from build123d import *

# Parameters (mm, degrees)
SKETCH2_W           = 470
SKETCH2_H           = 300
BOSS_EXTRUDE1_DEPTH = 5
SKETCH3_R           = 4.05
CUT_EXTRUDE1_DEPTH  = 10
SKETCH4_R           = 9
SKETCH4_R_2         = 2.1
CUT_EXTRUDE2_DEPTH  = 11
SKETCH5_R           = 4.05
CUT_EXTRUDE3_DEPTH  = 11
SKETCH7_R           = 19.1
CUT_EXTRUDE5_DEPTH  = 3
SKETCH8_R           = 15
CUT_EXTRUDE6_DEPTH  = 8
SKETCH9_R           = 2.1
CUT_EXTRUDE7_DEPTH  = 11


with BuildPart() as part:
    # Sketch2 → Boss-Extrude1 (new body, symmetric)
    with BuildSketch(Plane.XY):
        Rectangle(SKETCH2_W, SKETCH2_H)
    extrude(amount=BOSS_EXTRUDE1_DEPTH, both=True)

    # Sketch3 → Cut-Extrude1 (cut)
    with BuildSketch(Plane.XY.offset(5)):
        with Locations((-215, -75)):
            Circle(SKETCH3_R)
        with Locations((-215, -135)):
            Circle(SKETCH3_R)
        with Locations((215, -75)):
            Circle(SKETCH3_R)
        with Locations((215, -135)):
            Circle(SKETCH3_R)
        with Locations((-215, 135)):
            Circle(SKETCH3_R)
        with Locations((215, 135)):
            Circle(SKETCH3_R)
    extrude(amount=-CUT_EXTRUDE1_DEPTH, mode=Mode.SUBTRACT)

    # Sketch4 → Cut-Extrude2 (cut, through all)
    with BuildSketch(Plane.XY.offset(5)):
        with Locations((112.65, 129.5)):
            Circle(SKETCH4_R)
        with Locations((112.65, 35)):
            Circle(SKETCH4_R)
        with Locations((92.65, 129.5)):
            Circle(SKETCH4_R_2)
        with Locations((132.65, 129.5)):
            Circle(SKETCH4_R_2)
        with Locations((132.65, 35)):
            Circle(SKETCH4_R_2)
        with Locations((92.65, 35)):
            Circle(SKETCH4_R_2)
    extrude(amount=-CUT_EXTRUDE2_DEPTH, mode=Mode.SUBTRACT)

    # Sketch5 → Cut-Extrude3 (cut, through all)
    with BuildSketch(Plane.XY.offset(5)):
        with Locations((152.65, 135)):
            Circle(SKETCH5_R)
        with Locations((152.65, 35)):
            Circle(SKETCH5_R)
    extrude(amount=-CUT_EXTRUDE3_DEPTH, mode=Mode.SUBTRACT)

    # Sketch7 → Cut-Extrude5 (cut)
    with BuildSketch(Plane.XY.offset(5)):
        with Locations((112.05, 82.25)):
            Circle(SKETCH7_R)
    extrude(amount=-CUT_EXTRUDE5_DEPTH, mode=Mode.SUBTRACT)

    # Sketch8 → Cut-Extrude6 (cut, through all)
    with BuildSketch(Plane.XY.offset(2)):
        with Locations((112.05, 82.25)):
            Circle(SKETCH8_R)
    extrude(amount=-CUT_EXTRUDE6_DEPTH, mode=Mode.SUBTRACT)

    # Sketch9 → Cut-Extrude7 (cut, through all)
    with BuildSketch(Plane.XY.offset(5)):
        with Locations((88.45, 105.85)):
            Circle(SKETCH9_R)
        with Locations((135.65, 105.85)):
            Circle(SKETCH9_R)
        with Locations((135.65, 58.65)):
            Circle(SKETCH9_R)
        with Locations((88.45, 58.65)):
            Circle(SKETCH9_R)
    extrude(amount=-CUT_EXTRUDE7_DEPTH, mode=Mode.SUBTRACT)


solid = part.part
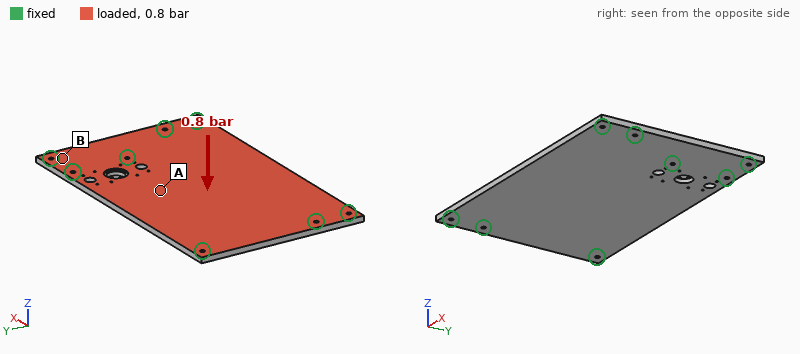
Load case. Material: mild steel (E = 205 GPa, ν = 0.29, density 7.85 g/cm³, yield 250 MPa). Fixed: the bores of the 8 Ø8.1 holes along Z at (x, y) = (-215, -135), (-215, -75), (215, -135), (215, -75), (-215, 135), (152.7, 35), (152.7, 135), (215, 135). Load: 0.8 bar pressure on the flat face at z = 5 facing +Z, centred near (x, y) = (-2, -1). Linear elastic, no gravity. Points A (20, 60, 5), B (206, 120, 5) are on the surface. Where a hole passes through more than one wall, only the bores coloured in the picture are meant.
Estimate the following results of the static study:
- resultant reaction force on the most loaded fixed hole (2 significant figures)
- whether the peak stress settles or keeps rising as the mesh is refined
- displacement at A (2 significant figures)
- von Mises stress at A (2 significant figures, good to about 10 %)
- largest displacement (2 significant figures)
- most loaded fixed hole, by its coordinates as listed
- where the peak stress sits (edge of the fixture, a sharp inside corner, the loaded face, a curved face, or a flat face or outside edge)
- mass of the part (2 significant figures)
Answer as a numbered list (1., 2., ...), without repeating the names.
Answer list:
1. 3.5 kN
2. keeps rising
3. 0.28 mm
4. 26 MPa
5. 0.43 mm
6. (152.7, 35)
7. edge of the fixture
8. 11 kg
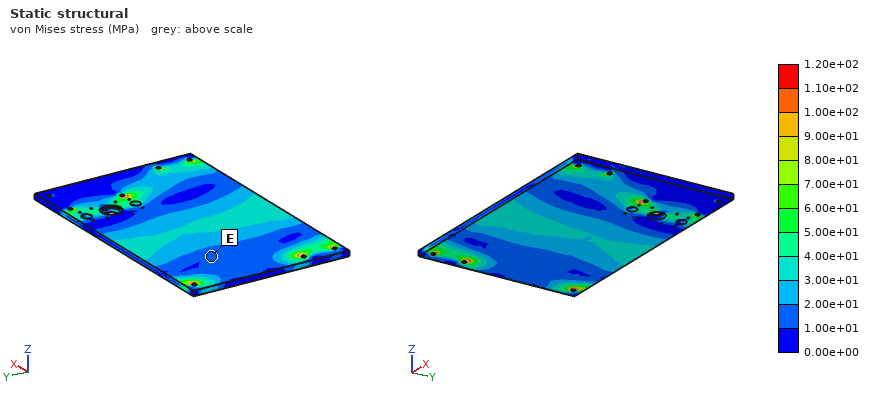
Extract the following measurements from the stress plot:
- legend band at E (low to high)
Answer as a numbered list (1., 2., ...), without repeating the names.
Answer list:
1. 1.00e+01 to 2.00e+01 MPa
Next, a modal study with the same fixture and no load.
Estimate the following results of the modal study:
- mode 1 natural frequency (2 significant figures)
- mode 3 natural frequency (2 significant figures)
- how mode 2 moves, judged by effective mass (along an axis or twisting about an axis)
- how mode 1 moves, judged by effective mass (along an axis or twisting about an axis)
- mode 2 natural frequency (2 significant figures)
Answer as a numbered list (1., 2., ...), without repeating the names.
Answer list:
1. 300 Hz
2. 790 Hz
3. twisting about X
4. along Z
5. 430 Hz
